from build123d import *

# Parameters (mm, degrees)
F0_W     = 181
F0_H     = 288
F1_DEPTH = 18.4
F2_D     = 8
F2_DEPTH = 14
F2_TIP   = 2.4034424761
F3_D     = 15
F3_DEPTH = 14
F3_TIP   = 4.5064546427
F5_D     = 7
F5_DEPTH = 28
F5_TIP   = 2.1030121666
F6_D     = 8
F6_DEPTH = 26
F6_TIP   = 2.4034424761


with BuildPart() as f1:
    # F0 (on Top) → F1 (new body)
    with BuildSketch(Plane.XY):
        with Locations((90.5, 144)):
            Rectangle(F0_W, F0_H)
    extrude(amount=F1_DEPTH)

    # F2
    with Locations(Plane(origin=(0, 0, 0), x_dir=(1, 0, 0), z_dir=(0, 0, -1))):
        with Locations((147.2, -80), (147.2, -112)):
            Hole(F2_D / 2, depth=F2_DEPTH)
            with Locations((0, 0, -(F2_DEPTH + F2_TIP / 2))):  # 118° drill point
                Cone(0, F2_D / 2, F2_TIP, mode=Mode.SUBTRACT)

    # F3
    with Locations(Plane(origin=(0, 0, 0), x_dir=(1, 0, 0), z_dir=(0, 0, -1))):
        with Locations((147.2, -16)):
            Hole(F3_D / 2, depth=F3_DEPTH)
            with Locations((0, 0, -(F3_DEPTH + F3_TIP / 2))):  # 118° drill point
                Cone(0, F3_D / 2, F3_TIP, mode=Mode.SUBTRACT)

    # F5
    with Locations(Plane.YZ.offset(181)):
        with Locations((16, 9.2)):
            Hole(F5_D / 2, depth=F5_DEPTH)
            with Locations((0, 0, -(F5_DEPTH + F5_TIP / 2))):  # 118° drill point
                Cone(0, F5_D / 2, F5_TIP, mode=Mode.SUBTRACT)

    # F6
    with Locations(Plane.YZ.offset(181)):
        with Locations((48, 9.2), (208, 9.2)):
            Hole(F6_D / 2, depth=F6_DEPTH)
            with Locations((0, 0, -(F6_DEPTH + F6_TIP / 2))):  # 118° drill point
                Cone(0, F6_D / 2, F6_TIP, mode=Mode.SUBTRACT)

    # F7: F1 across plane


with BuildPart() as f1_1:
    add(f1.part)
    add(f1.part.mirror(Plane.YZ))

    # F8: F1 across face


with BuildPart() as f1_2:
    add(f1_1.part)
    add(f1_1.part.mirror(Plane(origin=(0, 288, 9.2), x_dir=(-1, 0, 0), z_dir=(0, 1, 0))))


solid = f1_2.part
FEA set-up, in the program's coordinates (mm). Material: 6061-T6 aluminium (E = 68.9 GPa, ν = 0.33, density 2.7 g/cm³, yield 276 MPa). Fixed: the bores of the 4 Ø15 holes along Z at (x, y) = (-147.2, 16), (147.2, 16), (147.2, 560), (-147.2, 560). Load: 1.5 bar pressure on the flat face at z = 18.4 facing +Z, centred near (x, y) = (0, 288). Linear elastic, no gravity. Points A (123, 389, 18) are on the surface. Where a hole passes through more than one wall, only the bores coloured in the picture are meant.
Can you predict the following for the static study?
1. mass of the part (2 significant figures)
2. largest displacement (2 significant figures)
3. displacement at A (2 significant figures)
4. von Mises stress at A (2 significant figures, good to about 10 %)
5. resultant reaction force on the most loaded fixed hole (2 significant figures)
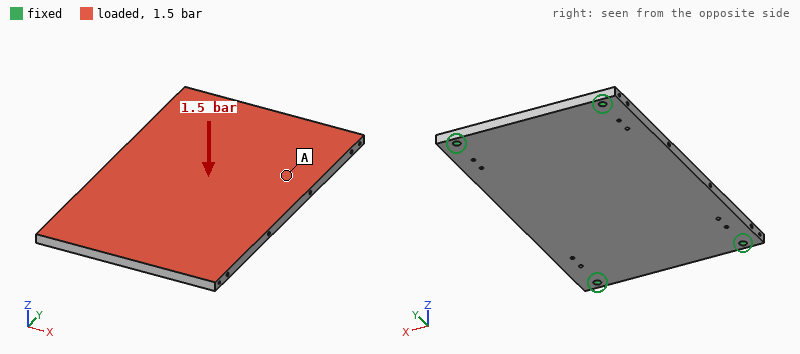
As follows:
10 kg
1.6 mm
1.2 mm
31 MPa
8.0 kN
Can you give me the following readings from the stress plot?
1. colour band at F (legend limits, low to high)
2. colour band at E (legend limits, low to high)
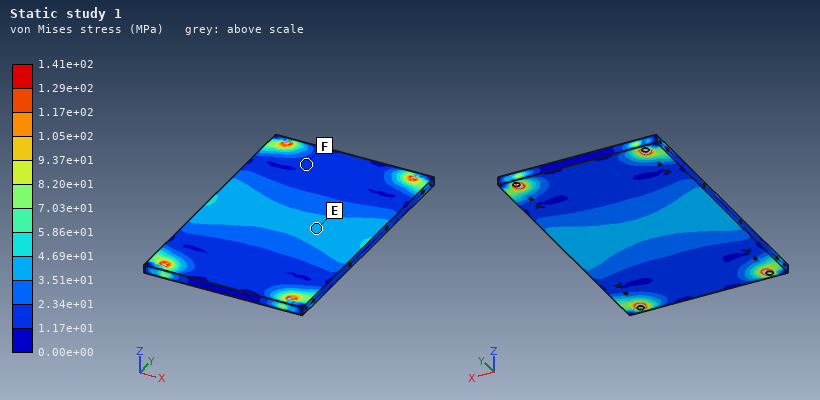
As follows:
1.17e+01 to 2.34e+01 MPa
3.51e+01 to 4.69e+01 MPa
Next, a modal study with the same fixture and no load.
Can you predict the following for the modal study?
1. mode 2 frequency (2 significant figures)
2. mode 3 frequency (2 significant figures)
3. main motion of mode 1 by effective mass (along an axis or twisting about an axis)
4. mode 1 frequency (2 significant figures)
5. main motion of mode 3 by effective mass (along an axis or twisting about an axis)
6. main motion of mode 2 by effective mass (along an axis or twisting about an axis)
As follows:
430 Hz
690 Hz
along Z
250 Hz
twisting about X
twisting about Y
